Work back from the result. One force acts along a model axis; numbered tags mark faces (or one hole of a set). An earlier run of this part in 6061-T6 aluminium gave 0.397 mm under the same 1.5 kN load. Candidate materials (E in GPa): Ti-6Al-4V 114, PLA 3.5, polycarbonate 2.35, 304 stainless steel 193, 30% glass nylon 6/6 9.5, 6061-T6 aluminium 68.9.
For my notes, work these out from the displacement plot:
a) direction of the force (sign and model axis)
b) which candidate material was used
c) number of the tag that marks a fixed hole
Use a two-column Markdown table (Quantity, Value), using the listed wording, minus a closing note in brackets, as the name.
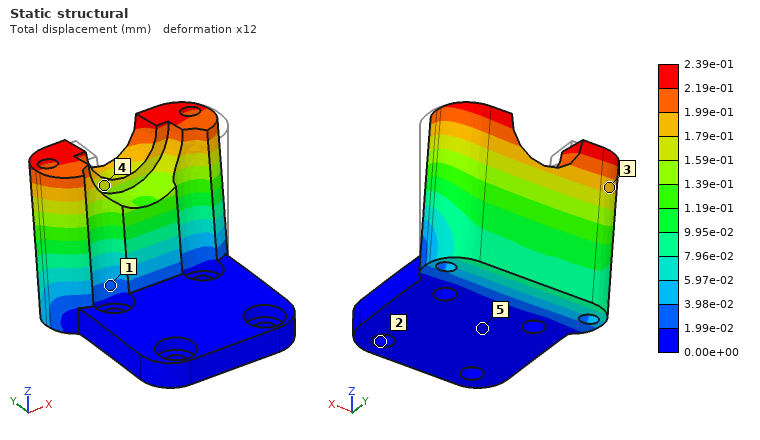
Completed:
| Quantity | Value |
|---|---|
| direction of the force | +Y |
| which candidate material was used | Ti-6Al-4V |
| number of the tag that marks a fixed hole | 2 |
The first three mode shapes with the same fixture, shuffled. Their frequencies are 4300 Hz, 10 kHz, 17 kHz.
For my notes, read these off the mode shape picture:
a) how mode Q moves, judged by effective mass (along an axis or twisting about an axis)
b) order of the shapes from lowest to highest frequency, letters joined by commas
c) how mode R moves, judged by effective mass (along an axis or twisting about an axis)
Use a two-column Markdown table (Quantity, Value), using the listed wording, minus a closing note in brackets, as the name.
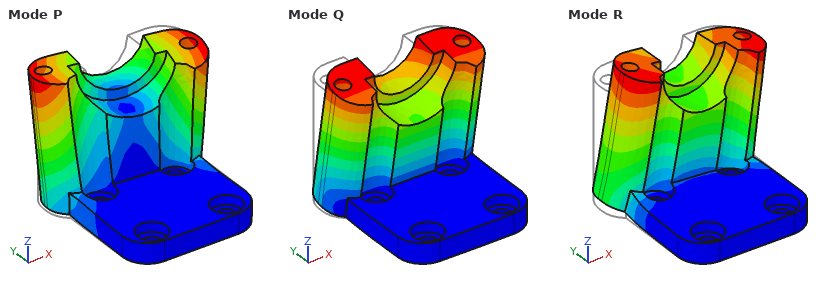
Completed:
| Quantity | Value |
|---|---|
| how mode Q moves, judged by effective mass | along Y |
| order of the shapes from lowest to highest frequency, letters joined by commas | Q, R, P |
| how mode R moves, judged by effective mass | along X |
